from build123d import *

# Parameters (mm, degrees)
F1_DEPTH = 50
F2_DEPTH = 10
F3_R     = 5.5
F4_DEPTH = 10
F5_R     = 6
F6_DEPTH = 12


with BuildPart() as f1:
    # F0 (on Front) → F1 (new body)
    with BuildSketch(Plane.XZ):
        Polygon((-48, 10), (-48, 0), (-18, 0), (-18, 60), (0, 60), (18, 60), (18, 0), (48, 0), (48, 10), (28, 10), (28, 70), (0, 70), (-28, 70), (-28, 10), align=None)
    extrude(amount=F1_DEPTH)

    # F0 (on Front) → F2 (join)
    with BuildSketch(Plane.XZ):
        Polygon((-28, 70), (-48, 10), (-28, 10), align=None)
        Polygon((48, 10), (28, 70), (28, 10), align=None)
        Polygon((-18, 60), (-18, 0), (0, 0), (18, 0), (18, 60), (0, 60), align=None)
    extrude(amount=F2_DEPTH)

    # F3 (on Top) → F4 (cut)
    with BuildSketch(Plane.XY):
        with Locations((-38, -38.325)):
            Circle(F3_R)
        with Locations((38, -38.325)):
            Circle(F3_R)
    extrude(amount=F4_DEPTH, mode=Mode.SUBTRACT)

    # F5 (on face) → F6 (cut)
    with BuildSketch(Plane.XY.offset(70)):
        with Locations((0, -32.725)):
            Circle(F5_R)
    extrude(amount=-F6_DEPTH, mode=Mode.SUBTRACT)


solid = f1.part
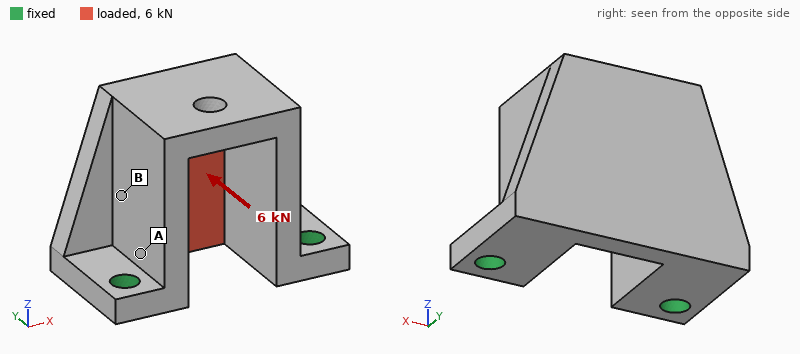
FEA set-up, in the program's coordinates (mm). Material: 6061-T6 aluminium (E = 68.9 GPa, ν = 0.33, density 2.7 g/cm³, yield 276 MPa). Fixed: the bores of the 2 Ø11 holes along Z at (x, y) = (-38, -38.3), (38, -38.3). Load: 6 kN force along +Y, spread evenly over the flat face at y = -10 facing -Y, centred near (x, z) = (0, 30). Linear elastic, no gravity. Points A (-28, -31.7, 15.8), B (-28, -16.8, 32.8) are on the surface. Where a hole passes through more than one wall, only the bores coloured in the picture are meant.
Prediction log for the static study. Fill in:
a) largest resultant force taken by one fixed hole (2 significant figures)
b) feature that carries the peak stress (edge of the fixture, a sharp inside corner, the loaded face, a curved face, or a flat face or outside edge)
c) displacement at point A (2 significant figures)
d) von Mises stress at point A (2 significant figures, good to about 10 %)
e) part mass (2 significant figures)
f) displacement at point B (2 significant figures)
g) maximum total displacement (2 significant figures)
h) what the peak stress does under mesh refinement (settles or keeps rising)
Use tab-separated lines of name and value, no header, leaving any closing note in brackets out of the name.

largest resultant force taken by one fixed hole	3.2 kN
feature that carries the peak stress	edge of the fixture
displacement at point A	0.034 mm
von Mises stress at point A	26 MPa
part mass	370 g
displacement at point B	0.093 mm
maximum total displacement	0.20 mm
what the peak stress does under mesh refinement	keeps rising
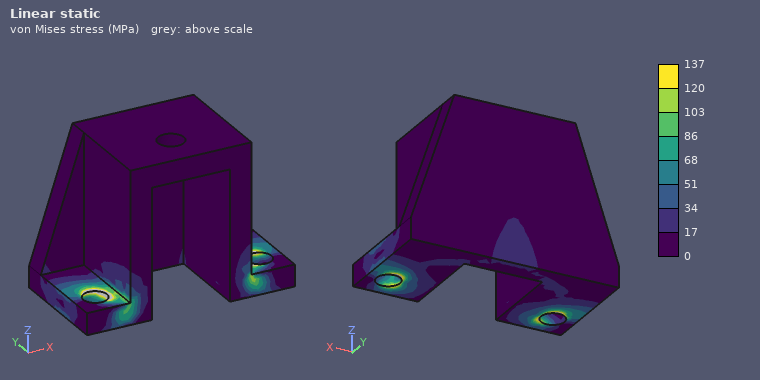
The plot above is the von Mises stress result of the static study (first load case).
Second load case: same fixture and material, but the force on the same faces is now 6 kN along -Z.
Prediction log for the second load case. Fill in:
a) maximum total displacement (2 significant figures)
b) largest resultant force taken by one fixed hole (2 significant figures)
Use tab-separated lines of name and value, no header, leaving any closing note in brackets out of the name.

maximum total displacement	0.20 mm
largest resultant force taken by one fixed hole	3.0 kN
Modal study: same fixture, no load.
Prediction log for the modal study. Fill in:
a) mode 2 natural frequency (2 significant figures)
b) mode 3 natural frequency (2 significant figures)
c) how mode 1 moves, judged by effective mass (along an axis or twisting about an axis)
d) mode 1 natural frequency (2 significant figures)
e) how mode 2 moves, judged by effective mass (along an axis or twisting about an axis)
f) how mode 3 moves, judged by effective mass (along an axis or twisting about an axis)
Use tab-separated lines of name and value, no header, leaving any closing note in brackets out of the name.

mode 2 natural frequency	2400 Hz
mode 3 natural frequency	5400 Hz
how mode 1 moves, judged by effective mass	along Y
mode 1 natural frequency	1500 Hz
how mode 2 moves, judged by effective mass	along X
how mode 3 moves, judged by effective mass	along X
